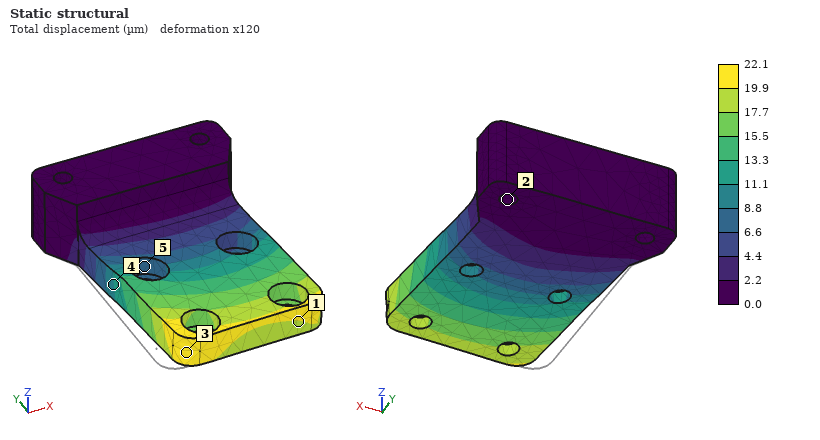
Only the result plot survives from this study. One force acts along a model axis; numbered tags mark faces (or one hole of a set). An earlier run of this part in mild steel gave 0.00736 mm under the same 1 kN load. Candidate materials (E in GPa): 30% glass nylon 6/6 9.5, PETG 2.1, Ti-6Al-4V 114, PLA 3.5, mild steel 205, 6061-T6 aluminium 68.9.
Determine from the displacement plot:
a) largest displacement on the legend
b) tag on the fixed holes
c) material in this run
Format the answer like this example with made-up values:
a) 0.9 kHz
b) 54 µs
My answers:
a) 22.1 µm
b) 2
c) 6061-T6 aluminium
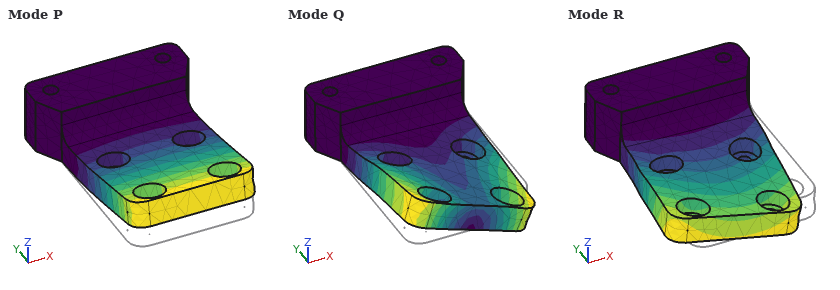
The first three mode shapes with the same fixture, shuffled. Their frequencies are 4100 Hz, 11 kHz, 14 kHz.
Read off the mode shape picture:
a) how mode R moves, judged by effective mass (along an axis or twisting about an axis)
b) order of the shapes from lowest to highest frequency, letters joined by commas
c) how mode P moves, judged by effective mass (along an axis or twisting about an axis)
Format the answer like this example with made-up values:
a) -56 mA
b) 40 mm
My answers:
a) along X
b) P, Q, R
c) along Z
